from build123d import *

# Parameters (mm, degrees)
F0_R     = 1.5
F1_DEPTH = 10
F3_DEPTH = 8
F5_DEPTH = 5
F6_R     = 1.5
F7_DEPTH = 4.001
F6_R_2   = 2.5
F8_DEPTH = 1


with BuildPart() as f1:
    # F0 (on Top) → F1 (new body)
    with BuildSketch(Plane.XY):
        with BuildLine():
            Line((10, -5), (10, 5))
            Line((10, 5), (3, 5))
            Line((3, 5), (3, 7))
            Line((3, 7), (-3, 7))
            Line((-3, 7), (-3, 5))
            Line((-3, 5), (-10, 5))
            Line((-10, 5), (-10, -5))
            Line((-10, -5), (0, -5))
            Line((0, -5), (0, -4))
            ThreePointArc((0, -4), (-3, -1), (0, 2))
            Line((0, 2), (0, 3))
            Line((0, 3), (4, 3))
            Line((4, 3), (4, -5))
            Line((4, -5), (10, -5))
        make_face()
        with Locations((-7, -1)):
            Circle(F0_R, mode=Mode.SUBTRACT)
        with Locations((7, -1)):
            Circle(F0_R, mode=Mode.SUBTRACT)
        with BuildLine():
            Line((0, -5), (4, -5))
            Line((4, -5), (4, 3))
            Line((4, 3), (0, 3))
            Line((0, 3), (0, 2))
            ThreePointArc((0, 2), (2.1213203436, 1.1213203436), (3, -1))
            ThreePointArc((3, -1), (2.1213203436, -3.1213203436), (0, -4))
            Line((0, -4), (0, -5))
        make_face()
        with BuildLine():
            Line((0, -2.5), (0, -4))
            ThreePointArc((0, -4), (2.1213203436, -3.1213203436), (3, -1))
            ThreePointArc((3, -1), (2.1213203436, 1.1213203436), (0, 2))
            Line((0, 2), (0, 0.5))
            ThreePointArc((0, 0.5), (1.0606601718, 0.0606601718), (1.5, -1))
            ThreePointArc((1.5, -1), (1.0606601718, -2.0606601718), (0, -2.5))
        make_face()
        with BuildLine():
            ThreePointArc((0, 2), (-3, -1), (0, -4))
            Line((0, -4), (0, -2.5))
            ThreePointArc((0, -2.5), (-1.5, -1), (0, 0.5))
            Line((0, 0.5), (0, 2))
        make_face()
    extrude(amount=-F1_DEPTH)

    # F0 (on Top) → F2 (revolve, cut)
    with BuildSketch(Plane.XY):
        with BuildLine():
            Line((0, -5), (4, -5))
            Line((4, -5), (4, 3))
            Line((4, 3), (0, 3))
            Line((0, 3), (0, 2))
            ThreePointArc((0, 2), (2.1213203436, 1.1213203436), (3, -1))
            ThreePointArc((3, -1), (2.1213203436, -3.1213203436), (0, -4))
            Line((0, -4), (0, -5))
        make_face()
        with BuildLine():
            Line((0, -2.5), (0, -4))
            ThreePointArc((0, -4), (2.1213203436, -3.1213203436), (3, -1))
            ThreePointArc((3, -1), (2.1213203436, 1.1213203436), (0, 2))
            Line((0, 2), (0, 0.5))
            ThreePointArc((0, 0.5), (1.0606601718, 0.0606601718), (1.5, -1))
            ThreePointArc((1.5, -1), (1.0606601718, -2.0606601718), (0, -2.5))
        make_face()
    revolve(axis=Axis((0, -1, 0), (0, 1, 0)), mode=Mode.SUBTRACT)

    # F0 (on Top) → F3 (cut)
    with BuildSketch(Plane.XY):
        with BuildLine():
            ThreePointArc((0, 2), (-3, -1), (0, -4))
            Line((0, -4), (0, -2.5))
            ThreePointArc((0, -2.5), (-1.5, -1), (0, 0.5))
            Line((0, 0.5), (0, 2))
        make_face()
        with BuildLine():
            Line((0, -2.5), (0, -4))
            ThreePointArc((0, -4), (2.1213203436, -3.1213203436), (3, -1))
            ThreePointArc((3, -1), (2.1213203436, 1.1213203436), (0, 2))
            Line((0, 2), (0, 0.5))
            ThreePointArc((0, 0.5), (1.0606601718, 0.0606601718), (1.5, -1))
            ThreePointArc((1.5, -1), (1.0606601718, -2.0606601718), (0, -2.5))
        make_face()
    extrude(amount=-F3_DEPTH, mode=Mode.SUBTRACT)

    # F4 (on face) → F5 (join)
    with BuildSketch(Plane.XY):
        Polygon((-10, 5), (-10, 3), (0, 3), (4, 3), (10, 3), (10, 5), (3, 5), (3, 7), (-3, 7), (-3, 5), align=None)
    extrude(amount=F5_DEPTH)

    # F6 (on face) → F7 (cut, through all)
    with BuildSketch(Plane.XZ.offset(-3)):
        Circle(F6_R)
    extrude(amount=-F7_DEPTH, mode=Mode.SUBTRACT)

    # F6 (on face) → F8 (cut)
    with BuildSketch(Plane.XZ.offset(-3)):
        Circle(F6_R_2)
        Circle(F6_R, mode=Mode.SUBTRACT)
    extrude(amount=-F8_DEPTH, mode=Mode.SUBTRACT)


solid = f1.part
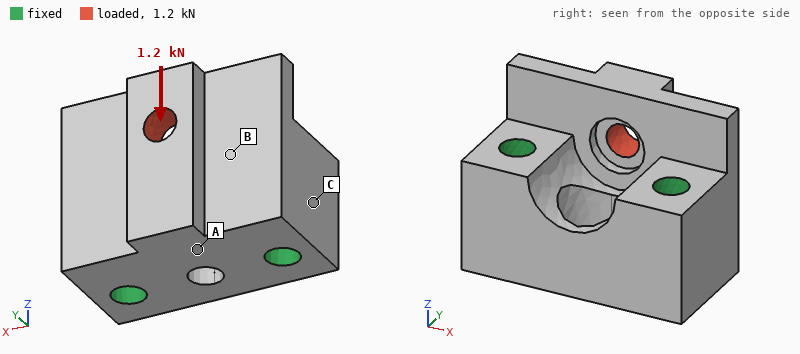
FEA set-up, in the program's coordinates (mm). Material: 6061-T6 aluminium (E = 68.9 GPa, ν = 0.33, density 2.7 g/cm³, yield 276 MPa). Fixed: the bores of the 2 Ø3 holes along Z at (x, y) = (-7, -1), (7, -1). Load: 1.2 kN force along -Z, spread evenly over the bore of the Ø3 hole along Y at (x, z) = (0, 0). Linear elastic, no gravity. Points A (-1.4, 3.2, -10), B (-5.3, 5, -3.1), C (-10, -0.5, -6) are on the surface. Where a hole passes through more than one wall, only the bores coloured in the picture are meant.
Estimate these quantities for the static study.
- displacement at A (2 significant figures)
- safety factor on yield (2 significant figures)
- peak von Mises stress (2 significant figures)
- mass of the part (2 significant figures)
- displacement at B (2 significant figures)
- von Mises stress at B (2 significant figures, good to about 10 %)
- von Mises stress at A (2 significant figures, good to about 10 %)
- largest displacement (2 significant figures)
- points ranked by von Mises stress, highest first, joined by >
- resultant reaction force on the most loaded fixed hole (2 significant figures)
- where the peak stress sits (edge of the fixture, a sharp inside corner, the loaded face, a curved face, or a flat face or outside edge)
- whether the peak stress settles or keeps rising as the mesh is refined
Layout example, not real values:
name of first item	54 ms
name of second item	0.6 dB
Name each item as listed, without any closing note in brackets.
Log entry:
displacement at A	4.2 µm
safety factor on yield	2.3
peak von Mises stress	120 MPa
mass of the part	5.0 g
displacement at B	3.2 µm
von Mises stress at B	39 MPa
von Mises stress at A	22 MPa
largest displacement	21 µm
points ranked by von Mises stress, highest first, joined by >	B > A > C
resultant reaction force on the most loaded fixed hole	600 N
where the peak stress sits	the loaded face
whether the peak stress settles or keeps rising as the mesh is refined	settles
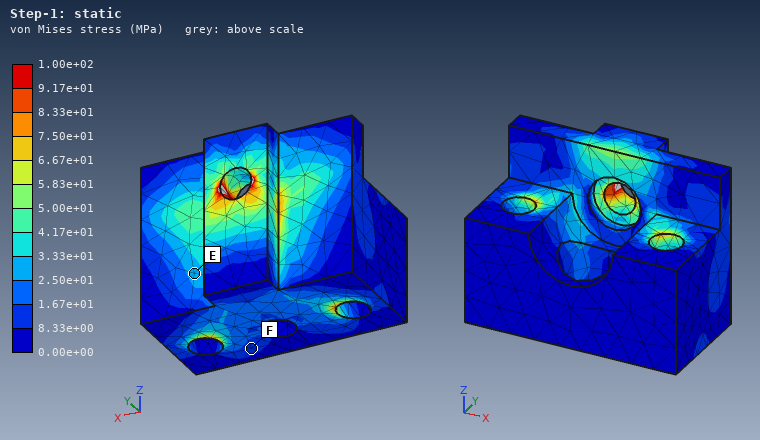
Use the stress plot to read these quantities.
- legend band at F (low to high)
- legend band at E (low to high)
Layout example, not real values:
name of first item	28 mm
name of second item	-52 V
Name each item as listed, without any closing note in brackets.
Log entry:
legend band at F	8.33e+00 to 1.67e+01 MPa
legend band at E	2.50e+01 to 3.33e+01 MPa
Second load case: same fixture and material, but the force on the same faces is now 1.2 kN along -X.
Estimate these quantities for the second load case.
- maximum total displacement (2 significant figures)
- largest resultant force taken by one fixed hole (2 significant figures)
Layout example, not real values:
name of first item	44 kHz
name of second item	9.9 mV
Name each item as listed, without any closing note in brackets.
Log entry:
maximum total displacement	11 µm
largest resultant force taken by one fixed hole	760 N
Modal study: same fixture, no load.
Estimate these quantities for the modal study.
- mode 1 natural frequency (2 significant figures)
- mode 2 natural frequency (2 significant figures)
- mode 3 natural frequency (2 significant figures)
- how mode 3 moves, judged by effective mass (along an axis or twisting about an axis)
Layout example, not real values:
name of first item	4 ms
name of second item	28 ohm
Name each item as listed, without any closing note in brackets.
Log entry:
mode 1 natural frequency	35 kHz
mode 2 natural frequency	49 kHz
mode 3 natural frequency	61 kHz
how mode 3 moves, judged by effective mass	along X
